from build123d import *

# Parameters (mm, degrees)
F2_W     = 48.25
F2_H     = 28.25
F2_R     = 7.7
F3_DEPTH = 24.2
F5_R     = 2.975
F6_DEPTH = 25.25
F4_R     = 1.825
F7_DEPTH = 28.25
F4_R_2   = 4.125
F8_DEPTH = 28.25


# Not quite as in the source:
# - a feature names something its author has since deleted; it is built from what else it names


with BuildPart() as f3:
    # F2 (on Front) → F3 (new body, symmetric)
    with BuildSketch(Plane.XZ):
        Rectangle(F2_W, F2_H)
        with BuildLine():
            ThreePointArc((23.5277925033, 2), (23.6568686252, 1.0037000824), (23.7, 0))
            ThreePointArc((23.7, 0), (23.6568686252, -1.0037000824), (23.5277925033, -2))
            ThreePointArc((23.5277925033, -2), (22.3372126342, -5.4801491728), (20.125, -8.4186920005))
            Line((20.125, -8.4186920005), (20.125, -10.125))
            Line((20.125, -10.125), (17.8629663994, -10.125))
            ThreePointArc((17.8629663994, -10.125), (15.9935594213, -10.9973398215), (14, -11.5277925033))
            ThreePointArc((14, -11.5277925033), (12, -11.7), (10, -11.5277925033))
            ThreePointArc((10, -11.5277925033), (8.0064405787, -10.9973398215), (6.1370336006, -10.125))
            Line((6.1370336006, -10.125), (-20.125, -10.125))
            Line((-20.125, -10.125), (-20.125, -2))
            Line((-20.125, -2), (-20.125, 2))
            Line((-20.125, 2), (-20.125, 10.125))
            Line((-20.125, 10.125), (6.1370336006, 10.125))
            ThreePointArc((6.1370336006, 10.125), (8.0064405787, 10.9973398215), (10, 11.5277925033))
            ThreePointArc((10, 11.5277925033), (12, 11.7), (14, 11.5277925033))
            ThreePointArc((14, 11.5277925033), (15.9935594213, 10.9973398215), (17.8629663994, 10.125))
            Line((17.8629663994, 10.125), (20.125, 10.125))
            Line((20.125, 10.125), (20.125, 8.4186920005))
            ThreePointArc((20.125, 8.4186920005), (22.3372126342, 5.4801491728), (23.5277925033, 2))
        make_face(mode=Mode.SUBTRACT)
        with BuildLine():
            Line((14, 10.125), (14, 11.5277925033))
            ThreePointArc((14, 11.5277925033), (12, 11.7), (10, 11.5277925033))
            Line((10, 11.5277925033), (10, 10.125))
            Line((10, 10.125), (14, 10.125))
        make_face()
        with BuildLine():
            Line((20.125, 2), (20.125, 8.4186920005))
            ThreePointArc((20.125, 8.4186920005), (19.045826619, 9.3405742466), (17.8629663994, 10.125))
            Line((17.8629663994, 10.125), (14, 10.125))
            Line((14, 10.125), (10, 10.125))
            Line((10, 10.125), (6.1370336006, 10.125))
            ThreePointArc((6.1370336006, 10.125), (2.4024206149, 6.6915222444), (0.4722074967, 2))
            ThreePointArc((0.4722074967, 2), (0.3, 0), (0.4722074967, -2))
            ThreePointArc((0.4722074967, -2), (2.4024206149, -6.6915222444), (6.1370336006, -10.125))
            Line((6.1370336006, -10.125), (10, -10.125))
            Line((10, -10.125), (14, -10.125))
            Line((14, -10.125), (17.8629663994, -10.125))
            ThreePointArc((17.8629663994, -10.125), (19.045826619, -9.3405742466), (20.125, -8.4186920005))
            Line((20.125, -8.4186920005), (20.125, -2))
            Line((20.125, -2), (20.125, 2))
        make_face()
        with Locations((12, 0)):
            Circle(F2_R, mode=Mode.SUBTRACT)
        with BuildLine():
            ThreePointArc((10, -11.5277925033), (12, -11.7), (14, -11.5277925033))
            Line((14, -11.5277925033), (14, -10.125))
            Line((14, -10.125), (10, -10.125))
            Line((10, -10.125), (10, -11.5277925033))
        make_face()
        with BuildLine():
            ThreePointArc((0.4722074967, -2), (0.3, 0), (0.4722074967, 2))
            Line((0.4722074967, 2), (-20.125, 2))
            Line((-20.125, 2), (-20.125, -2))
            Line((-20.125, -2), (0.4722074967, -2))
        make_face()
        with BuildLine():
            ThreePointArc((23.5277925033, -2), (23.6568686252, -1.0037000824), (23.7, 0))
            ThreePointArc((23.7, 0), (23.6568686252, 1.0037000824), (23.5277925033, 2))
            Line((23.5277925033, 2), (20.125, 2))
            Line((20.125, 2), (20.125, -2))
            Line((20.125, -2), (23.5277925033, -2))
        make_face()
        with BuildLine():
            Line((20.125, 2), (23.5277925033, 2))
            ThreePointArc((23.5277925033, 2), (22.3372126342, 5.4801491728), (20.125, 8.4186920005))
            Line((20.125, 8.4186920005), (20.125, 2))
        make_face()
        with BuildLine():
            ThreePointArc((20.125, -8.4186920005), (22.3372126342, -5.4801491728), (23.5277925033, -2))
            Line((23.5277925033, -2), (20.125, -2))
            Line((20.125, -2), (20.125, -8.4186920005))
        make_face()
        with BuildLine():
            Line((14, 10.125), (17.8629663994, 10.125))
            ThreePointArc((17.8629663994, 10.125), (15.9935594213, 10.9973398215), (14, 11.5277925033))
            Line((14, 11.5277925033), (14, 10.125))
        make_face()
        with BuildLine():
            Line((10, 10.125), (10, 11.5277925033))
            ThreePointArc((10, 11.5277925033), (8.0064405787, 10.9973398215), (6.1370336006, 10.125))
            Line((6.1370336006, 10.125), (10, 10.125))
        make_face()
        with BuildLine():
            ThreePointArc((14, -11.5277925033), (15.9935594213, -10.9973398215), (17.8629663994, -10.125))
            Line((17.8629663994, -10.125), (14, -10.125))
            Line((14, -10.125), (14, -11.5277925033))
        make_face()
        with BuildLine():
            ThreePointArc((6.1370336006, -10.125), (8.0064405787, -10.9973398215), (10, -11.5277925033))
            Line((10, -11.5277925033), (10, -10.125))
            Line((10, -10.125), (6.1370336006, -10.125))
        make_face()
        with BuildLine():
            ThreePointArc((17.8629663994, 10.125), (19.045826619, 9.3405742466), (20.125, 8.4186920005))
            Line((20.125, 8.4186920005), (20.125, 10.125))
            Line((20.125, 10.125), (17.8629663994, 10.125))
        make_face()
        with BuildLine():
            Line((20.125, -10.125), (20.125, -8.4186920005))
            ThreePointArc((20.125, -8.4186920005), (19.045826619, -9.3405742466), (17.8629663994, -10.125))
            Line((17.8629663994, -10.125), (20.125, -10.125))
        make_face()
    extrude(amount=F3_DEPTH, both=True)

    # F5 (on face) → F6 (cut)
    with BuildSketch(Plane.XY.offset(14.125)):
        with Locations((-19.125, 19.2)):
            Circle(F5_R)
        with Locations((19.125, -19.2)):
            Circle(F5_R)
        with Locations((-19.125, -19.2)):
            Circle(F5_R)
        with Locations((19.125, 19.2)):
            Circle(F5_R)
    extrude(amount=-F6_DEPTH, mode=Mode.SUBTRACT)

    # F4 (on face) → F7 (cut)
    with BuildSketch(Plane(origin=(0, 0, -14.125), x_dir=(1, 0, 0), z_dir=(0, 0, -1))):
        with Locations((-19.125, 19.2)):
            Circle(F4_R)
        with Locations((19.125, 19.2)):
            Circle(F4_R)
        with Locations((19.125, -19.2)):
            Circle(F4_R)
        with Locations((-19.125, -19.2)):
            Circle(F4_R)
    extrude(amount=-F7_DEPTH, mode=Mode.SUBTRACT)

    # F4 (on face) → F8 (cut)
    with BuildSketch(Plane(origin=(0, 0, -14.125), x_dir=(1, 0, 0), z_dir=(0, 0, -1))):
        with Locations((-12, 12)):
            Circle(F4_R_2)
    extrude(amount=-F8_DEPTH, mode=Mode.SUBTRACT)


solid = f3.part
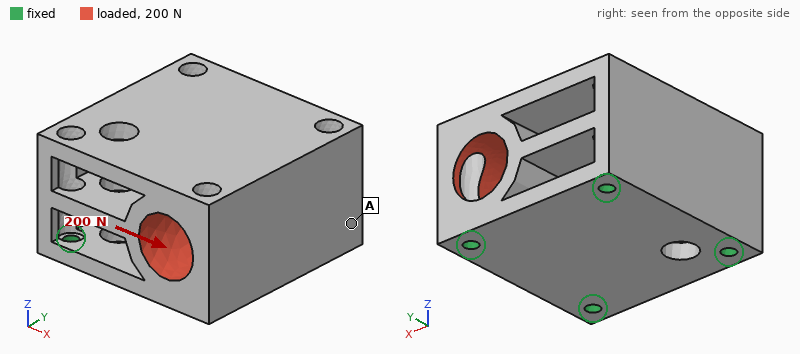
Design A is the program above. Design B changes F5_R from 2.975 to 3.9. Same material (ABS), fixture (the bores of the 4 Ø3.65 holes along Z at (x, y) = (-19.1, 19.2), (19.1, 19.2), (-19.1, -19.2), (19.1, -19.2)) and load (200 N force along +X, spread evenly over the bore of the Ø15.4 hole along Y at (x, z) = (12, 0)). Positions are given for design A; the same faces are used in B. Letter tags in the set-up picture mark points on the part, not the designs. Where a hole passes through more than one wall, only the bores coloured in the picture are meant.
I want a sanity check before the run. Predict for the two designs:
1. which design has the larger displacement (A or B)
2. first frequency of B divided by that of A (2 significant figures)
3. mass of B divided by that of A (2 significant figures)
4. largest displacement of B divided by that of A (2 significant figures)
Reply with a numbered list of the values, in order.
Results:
1. B
2. 0.98
3. 0.96
4. 1.1
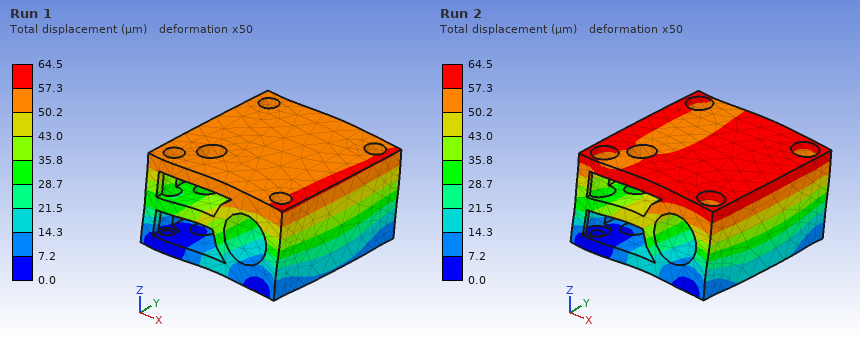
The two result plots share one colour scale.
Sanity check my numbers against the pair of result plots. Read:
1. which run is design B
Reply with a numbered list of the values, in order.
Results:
1. Run 2
